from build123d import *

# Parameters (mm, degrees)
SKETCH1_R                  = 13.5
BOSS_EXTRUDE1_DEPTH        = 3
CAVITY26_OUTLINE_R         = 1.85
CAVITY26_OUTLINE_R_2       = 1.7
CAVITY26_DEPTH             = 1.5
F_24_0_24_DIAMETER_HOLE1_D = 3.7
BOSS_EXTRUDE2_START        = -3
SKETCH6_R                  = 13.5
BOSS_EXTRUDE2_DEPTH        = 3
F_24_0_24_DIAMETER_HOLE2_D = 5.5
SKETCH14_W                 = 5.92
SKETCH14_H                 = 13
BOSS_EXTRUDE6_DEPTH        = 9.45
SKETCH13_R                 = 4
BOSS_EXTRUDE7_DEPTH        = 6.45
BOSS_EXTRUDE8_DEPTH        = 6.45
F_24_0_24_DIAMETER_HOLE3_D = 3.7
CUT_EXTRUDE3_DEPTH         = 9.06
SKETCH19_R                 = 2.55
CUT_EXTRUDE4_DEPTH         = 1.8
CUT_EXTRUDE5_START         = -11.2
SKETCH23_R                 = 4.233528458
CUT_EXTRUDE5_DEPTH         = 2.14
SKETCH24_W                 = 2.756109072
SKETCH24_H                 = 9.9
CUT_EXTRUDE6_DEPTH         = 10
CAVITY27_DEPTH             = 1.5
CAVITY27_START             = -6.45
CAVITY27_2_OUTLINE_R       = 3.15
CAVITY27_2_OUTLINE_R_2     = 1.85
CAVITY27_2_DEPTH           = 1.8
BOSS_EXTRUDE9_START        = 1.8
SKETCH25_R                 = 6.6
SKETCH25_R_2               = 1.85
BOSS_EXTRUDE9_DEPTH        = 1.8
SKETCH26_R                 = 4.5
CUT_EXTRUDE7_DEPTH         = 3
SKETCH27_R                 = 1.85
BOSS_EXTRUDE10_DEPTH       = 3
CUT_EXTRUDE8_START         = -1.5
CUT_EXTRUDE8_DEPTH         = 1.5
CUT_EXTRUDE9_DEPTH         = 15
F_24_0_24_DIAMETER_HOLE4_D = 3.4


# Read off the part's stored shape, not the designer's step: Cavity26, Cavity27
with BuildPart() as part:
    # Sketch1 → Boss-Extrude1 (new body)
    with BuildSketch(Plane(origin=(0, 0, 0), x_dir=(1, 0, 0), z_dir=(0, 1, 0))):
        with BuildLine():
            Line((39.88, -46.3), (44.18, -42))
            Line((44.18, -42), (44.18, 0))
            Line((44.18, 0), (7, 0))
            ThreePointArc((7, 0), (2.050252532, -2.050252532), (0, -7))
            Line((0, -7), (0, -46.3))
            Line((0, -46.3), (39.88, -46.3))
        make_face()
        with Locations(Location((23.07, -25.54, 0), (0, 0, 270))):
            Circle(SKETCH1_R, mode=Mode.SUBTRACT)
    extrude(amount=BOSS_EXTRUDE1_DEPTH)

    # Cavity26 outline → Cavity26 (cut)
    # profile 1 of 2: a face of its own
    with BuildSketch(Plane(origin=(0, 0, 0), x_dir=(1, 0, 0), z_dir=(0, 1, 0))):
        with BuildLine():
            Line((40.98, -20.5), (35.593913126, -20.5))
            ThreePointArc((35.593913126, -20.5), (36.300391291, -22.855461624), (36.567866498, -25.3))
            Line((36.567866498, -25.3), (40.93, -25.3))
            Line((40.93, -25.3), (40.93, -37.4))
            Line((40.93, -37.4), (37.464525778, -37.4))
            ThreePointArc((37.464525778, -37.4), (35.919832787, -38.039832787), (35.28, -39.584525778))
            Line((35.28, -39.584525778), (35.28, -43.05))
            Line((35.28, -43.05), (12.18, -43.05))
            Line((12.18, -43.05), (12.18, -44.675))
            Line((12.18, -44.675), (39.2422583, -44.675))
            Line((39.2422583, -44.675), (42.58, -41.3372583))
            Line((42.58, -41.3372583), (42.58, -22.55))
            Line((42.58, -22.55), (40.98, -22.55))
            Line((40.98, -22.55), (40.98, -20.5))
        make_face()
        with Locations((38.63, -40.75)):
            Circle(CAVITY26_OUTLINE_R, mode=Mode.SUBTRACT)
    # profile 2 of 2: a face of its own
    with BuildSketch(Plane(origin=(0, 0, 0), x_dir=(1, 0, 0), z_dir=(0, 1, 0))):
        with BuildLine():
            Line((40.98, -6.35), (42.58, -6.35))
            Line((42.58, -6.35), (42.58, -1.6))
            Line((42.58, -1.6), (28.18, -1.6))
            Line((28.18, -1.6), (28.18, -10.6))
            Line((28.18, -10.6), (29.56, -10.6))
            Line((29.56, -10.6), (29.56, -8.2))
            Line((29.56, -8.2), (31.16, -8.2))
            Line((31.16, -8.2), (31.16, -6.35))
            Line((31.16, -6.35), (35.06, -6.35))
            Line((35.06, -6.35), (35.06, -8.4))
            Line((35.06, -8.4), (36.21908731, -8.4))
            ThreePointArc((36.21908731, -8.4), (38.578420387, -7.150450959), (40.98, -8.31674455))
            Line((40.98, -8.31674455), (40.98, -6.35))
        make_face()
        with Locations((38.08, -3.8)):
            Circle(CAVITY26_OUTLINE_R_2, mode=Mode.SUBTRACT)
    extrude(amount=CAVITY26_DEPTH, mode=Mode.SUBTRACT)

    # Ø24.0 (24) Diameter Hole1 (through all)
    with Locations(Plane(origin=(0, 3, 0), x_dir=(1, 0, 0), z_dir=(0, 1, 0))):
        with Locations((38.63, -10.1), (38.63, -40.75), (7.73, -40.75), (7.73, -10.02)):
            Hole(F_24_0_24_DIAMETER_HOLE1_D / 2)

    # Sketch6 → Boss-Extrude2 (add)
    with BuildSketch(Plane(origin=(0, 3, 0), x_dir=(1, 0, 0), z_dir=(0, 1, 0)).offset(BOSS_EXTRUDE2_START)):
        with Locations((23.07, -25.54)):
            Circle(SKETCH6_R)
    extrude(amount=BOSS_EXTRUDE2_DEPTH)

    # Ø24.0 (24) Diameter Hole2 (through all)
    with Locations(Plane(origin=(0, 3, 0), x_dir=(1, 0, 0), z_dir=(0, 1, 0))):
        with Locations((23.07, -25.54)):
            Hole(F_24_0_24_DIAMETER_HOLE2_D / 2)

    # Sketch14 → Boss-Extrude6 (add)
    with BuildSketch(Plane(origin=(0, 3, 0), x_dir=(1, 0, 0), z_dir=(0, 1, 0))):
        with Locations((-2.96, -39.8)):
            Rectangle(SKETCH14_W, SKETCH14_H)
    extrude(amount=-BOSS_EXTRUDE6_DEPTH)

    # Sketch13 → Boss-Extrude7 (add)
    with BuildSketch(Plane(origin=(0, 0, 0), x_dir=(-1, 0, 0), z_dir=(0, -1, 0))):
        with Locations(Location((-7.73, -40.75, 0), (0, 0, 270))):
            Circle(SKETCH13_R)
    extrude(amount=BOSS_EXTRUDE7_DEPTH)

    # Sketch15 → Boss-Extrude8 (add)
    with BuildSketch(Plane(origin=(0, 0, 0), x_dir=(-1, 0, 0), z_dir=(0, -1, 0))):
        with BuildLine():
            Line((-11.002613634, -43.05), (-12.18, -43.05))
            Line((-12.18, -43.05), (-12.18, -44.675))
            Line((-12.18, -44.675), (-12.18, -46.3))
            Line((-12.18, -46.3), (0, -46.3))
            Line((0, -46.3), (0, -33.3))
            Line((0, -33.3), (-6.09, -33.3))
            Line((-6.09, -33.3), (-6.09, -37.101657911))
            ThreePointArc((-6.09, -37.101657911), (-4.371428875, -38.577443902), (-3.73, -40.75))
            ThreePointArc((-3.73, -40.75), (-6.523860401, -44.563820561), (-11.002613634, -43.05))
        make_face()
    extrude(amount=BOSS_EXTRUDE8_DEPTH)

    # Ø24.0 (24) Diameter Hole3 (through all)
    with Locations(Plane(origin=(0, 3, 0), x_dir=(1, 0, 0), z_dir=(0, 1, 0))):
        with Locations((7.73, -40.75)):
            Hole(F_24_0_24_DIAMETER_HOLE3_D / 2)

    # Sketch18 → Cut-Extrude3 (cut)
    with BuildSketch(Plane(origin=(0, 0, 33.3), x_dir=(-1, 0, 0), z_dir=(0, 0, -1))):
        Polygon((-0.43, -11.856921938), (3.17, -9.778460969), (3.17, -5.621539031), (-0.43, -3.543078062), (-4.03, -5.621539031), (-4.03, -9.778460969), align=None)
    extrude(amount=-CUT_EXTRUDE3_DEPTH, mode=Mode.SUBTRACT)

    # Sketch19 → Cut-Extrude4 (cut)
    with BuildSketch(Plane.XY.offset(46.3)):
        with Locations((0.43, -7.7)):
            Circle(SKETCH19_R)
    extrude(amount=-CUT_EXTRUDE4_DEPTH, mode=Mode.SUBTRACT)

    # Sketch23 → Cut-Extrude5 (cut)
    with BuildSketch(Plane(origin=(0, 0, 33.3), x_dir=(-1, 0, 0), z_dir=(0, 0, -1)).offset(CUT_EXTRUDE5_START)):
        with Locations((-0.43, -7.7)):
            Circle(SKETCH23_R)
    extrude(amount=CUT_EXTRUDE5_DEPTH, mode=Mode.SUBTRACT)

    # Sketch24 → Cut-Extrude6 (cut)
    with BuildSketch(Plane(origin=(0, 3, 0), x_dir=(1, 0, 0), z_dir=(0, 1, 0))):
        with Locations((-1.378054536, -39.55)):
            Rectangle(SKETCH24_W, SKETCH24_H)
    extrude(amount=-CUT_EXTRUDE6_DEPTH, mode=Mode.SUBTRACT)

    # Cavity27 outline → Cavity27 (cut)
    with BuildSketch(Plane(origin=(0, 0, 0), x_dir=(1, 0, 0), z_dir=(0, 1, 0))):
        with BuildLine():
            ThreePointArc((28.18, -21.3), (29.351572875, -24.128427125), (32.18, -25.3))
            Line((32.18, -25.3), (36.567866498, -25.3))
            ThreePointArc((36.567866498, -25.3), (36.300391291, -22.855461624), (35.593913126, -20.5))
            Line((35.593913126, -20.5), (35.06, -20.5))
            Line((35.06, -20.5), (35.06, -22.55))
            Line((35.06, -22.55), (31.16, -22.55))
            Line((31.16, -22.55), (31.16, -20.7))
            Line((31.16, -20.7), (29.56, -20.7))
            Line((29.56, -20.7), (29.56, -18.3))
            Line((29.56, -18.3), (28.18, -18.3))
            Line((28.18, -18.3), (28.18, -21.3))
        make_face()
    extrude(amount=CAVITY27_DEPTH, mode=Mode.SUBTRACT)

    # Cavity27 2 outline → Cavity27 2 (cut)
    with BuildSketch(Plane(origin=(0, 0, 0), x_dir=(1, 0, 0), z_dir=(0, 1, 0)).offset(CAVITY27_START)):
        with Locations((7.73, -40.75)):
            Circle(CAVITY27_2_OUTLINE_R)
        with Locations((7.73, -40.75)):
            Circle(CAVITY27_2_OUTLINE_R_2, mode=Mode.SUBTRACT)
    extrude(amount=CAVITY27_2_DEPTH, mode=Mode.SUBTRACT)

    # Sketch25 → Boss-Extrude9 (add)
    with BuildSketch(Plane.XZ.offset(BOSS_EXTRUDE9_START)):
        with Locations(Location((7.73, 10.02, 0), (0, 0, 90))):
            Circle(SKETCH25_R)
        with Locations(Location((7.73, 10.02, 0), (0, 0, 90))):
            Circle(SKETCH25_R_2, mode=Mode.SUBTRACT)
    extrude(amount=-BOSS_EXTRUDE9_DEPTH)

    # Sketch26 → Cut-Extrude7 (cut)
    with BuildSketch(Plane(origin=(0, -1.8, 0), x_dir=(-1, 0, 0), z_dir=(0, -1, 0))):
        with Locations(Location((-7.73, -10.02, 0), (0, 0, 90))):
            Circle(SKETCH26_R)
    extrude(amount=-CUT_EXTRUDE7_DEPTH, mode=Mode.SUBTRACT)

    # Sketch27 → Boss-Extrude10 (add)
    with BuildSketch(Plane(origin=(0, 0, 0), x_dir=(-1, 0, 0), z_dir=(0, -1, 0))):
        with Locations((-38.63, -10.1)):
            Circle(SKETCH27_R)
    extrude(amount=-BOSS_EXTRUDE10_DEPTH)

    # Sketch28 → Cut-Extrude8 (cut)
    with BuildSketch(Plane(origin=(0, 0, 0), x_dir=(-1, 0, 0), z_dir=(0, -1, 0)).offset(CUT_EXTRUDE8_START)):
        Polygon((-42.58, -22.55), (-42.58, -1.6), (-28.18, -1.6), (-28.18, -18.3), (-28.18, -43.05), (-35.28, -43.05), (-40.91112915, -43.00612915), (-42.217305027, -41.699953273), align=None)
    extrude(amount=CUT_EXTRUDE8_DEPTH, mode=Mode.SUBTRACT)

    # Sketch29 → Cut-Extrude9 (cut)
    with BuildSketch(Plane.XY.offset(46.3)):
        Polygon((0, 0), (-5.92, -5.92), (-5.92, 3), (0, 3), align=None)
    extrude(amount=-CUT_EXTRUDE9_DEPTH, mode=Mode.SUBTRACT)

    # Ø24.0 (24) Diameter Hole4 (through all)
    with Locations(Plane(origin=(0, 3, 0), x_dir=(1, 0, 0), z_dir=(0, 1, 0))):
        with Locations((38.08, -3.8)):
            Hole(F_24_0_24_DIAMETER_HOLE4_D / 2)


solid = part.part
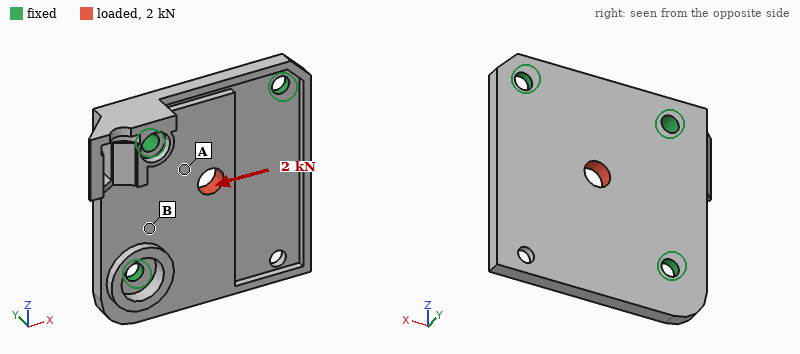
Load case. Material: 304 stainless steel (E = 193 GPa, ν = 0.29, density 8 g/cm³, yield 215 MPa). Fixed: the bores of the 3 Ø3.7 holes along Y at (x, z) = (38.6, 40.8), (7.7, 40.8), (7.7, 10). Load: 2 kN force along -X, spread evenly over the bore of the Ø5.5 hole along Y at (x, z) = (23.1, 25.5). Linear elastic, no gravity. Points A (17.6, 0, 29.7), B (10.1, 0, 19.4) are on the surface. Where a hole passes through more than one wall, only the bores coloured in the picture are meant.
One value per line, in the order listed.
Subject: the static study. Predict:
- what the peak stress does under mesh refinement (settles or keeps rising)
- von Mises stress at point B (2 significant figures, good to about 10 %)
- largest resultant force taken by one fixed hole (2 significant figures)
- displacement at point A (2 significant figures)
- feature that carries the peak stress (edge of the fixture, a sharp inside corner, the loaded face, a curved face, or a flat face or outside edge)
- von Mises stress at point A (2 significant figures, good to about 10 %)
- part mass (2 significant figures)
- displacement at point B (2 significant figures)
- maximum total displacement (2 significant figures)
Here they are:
keeps rising
12 MPa
900 N
2.4 µm
edge of the fixture
29 MPa
46 g
2.0 µm
4.9 µm
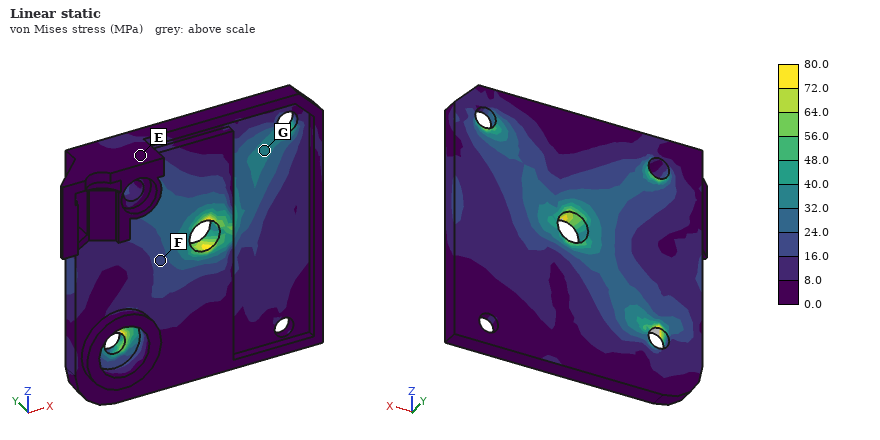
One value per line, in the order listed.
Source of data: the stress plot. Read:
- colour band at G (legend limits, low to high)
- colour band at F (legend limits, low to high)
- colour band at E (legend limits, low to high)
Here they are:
32.0 to 40.0 MPa
16.0 to 24.0 MPa
0.0 to 8.0 MPa
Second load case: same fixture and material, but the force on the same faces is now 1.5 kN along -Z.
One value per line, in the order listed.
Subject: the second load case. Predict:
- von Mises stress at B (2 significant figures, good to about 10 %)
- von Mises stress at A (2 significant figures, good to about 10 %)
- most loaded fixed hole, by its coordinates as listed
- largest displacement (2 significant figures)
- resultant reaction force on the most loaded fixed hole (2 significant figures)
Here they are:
9.9 MPa
22 MPa
(7.7, 40.8)
4.3 µm
680 N
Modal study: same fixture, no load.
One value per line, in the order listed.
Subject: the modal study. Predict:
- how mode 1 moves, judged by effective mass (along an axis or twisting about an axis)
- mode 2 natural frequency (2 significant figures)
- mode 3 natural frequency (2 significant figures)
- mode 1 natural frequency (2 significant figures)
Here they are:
along Y
7800 Hz
7900 Hz
2700 Hz
